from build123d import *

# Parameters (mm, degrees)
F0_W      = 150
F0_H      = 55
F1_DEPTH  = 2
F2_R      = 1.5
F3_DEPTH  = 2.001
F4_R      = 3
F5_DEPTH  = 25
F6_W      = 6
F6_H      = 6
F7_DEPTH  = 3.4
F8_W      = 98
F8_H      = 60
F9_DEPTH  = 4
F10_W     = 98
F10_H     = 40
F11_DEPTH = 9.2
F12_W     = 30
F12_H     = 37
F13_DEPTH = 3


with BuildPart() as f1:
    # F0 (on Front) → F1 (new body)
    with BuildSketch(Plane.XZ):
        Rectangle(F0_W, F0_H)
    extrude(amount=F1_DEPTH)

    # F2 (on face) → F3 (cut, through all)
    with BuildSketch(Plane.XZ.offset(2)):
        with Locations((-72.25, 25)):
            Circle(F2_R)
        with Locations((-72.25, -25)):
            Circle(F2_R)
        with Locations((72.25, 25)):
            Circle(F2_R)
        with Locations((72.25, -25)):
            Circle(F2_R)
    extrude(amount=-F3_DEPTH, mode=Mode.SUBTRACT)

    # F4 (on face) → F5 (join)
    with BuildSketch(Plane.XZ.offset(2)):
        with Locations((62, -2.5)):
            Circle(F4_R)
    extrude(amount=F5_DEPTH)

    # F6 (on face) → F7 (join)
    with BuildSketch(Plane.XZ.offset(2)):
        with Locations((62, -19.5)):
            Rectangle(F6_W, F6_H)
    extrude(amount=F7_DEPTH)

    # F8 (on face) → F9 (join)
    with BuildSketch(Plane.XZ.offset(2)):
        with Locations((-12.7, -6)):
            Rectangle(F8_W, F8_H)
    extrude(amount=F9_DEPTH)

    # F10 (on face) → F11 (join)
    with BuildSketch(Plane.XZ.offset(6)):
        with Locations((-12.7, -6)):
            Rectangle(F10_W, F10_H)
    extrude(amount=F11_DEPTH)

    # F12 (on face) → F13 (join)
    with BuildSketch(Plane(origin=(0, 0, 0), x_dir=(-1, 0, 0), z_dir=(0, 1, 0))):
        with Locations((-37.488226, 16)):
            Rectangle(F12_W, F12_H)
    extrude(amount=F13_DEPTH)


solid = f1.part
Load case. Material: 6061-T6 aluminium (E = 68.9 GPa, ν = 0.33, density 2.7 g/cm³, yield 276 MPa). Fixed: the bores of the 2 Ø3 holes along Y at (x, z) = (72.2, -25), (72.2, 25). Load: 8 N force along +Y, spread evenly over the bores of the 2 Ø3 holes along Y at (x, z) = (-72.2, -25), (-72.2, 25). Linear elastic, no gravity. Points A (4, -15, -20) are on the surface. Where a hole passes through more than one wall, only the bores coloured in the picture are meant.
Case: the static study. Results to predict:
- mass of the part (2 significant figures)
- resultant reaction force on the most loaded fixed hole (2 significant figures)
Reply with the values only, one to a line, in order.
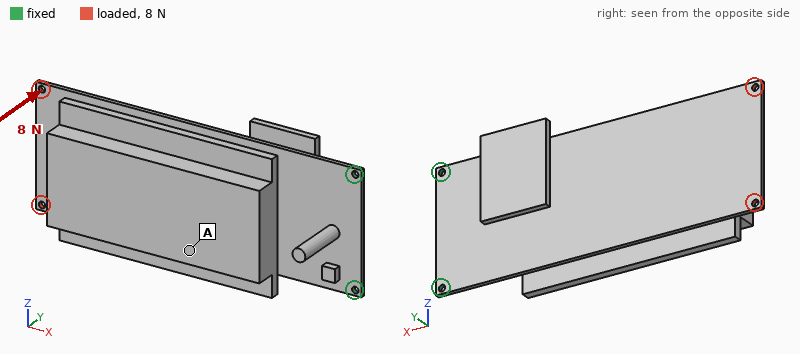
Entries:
220 g
7.0 N
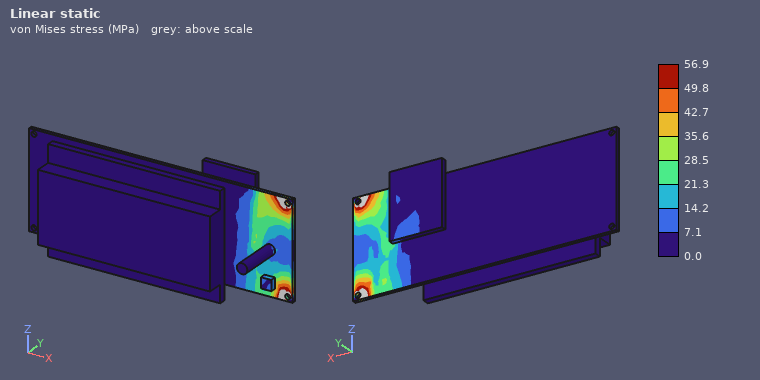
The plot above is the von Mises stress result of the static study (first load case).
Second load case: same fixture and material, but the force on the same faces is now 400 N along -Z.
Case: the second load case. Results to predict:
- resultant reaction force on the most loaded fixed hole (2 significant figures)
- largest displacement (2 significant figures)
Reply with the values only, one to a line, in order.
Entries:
1.2 kN
0.22 mm
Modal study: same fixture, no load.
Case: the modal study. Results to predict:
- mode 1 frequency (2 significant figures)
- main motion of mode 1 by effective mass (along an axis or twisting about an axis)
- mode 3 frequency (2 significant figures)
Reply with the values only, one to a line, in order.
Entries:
41 Hz
along Y
840 Hz
